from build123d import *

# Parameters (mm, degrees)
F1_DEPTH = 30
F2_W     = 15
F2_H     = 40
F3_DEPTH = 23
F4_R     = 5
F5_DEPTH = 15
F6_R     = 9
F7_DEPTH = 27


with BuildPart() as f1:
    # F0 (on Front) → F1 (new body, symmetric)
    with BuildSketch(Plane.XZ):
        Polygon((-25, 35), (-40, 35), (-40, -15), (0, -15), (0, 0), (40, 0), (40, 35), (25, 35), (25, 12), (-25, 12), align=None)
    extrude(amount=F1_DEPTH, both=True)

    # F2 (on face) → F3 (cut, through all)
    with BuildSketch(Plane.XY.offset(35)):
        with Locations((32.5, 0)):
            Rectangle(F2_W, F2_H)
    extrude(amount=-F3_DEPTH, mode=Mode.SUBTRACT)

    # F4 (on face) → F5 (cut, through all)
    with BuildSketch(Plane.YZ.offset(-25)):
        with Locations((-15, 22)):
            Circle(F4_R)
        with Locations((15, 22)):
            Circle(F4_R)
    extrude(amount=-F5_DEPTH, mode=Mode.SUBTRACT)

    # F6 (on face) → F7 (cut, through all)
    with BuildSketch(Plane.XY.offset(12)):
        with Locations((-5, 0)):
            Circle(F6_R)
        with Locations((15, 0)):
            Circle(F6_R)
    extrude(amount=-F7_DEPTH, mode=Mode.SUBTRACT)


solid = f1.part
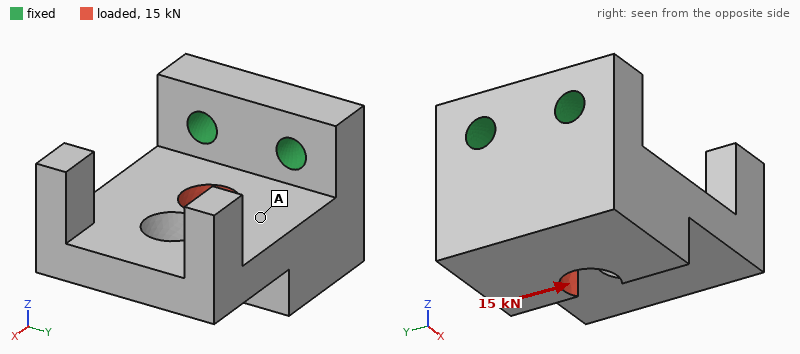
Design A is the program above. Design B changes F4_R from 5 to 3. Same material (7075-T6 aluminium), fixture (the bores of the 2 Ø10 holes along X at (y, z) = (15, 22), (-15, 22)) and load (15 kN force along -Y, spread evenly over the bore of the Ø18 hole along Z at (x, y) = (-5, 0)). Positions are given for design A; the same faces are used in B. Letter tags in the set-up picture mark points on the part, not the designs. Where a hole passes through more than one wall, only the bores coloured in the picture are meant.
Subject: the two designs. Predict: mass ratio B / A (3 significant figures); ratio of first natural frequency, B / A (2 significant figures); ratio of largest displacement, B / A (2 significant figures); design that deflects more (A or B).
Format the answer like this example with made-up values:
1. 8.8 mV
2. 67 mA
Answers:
1. 1.01
2. 0.93
3. 1.2
4. B
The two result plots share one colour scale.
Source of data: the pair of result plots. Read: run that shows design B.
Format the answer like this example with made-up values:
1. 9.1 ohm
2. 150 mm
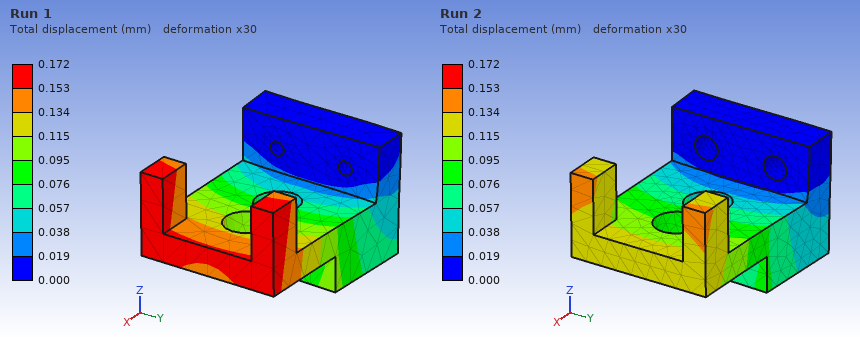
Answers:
1. Run 1
